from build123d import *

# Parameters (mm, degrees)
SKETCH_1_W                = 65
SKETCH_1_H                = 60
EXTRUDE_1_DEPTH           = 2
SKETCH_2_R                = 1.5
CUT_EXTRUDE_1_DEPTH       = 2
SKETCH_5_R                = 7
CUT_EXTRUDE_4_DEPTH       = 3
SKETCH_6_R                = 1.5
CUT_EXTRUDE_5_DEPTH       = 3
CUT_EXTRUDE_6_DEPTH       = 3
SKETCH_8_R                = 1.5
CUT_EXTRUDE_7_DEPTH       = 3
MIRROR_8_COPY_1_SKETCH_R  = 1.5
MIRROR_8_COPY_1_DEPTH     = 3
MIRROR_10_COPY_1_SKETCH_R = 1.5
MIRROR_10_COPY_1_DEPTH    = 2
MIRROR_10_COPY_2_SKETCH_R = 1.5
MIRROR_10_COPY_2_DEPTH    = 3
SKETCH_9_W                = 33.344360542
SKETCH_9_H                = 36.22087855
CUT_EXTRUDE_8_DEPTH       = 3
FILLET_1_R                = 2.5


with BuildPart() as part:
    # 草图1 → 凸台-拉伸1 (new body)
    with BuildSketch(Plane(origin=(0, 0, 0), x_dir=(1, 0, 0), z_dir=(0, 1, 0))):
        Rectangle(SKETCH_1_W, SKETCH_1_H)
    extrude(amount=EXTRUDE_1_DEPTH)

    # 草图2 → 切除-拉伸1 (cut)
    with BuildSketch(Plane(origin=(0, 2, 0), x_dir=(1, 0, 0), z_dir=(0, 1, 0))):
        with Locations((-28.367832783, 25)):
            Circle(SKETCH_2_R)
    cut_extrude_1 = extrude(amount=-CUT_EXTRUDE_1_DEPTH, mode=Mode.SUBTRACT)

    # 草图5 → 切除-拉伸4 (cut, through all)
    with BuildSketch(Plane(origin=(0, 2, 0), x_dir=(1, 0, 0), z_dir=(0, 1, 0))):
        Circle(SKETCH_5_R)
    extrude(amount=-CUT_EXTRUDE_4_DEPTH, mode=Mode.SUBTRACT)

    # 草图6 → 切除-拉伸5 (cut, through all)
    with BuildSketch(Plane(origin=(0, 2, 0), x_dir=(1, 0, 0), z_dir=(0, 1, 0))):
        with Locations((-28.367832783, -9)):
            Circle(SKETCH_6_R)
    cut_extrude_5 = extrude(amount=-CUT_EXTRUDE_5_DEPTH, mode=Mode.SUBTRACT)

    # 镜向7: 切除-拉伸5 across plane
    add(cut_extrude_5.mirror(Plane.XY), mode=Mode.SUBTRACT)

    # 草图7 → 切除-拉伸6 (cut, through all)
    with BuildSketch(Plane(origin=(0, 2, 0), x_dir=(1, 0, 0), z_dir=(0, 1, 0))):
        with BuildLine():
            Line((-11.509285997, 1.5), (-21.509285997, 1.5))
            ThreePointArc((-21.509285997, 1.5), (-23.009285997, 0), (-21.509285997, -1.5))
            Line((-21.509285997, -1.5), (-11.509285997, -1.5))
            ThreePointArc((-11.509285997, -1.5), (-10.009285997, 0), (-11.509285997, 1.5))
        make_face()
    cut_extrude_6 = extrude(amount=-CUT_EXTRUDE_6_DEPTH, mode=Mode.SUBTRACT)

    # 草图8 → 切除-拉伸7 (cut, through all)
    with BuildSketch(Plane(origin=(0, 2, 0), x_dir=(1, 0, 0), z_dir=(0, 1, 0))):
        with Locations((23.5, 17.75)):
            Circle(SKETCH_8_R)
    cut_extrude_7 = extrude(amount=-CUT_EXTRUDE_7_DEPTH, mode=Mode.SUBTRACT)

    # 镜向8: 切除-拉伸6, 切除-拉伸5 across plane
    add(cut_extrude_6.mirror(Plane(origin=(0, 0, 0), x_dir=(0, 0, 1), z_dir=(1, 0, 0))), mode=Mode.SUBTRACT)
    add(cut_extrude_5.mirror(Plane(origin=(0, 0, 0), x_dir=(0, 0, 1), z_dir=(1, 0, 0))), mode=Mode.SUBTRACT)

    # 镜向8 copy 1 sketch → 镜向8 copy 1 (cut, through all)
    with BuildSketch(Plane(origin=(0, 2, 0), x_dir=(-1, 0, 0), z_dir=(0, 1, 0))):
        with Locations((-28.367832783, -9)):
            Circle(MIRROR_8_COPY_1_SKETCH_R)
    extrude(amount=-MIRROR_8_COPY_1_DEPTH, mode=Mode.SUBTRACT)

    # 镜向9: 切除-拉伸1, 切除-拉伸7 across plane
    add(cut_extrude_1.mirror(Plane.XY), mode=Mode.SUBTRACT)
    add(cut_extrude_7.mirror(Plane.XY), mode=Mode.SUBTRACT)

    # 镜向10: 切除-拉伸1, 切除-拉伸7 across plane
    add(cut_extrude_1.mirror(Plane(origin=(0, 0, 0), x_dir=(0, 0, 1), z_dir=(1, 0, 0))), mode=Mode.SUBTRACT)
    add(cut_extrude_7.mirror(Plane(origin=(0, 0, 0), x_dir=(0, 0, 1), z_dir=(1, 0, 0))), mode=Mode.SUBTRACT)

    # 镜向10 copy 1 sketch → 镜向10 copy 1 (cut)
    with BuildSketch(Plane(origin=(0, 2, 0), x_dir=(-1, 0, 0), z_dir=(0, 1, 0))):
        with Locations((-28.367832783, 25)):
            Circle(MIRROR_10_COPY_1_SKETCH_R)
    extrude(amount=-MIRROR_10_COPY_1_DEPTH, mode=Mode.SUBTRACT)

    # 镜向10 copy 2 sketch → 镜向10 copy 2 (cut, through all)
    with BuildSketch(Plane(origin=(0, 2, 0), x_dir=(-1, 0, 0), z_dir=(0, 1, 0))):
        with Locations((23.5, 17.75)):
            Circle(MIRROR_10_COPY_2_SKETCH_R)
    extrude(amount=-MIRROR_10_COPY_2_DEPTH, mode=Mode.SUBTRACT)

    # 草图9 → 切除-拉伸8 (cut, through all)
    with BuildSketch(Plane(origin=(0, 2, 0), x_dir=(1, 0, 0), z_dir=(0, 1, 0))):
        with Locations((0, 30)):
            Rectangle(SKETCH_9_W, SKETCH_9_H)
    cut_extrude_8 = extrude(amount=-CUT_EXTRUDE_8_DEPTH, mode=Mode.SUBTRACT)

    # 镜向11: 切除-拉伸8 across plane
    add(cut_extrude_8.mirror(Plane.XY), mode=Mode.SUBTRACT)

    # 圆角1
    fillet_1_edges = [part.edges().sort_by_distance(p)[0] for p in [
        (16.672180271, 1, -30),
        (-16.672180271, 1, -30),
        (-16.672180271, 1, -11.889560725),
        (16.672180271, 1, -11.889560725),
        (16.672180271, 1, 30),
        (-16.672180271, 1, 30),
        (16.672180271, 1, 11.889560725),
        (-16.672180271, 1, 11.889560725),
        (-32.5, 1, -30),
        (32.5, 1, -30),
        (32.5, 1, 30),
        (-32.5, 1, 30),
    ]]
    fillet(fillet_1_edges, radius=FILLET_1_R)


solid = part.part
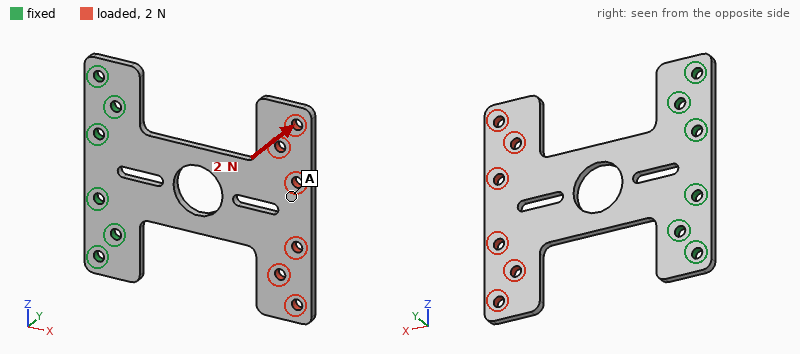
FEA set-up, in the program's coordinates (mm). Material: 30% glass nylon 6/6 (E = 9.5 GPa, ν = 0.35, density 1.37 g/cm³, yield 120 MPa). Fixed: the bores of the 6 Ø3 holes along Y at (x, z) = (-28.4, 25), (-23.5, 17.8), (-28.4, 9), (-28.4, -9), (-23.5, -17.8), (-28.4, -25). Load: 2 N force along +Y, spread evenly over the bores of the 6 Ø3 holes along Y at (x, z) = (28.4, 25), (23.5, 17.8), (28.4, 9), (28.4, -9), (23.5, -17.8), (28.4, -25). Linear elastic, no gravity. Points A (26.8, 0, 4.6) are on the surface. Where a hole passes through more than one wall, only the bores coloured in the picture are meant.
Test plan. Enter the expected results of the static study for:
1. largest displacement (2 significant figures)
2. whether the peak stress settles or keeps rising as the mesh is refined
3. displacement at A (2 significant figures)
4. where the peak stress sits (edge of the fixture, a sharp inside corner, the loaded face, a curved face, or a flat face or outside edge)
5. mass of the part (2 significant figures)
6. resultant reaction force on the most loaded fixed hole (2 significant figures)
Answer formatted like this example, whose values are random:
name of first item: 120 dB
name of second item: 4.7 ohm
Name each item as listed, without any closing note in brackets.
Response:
largest displacement: 0.91 mm
whether the peak stress settles or keeps rising as the mesh is refined: keeps rising
displacement at A: 0.76 mm
where the peak stress sits: a sharp inside corner
mass of the part: 6.5 g
resultant reaction force on the most loaded fixed hole: 2.9 N
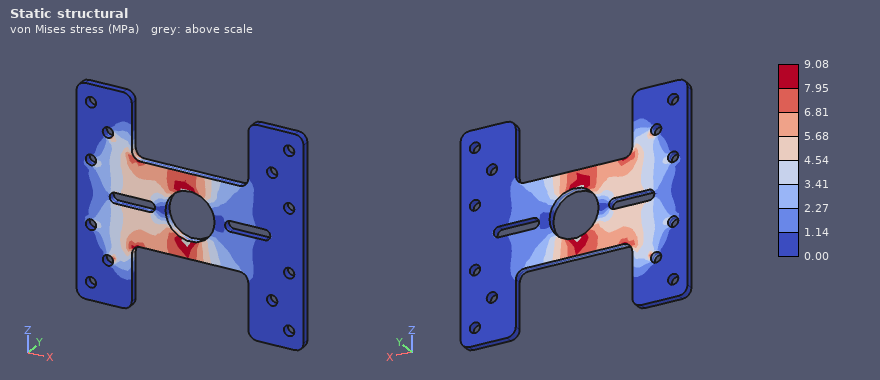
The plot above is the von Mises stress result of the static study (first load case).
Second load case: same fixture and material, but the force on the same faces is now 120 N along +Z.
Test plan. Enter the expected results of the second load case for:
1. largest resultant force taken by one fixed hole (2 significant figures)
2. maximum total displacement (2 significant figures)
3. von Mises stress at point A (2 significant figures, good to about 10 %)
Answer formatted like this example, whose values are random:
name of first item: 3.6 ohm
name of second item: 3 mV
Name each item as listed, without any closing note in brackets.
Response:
largest resultant force taken by one fixed hole: 120 N
maximum total displacement: 0.48 mm
von Mises stress at point A: 4.7 MPa
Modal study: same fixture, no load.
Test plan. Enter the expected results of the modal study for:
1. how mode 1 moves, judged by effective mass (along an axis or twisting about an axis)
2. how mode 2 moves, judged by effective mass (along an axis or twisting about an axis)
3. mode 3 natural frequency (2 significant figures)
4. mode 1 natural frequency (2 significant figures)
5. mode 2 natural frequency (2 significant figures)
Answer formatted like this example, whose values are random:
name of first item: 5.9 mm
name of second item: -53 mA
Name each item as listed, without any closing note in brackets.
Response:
how mode 1 moves, judged by effective mass: along Y
how mode 2 moves, judged by effective mass: twisting about X
mode 3 natural frequency: 1400 Hz
mode 1 natural frequency: 170 Hz
mode 2 natural frequency: 370 Hz
